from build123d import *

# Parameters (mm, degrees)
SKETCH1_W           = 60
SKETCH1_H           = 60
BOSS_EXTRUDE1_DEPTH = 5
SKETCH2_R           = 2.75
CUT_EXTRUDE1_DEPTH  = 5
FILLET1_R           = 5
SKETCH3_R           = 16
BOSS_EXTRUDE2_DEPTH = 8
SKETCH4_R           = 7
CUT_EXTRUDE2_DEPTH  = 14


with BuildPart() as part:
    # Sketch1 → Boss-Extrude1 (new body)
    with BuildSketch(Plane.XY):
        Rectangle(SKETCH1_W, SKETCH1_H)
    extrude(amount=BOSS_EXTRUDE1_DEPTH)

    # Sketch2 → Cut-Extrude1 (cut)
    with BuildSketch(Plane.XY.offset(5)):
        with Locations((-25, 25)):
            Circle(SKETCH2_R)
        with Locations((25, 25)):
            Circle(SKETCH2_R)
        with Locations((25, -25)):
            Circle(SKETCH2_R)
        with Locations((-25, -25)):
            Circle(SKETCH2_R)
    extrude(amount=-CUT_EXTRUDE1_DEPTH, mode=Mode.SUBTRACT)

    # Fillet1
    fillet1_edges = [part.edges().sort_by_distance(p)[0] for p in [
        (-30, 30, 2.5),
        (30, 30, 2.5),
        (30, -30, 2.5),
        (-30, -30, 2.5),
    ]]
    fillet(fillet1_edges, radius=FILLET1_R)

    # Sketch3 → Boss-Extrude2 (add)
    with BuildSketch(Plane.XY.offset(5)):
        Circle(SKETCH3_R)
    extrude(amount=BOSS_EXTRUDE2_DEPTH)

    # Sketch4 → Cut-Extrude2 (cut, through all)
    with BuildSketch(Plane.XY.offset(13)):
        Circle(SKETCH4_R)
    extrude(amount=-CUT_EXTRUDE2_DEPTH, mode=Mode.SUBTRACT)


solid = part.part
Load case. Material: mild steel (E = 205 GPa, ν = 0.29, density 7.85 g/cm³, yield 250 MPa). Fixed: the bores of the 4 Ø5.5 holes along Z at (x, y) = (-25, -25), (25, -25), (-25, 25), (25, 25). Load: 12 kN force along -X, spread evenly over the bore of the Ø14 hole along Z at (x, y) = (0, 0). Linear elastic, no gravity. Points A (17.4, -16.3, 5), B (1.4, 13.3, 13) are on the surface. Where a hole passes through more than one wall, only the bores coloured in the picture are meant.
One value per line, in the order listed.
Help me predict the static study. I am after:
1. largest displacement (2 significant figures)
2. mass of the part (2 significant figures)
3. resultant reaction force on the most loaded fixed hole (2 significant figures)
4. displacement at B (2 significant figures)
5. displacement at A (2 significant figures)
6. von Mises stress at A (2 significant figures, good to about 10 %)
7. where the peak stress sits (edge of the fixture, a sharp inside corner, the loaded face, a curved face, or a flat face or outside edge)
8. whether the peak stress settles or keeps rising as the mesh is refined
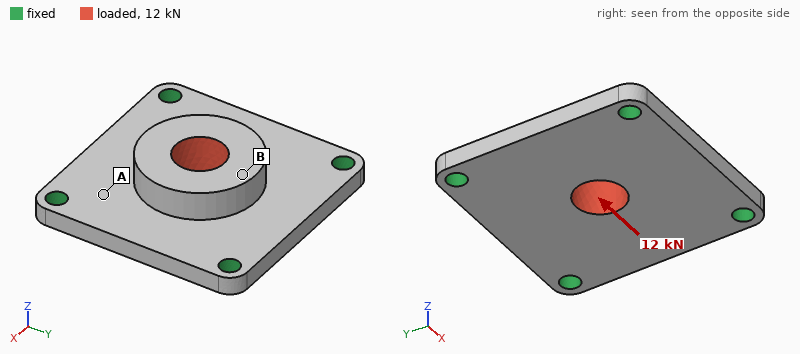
15 µm
170 g
3.4 kN
11 µm
5.0 µm
60 MPa
edge of the fixture
keeps rising
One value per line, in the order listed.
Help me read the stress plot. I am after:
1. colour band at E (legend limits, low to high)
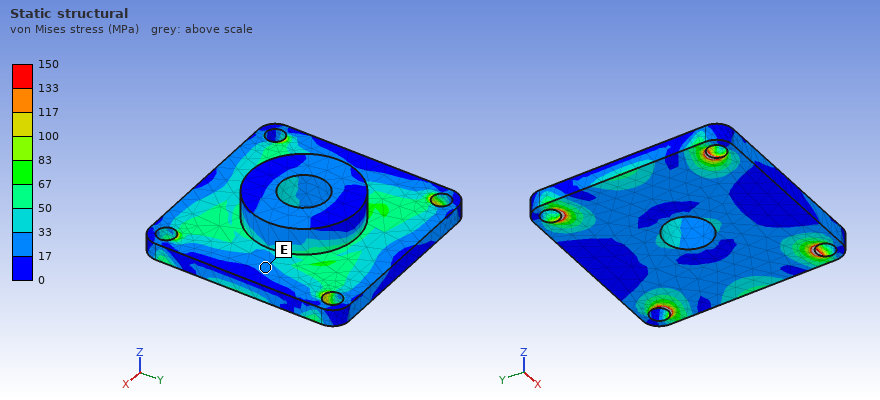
17 to 33 MPa
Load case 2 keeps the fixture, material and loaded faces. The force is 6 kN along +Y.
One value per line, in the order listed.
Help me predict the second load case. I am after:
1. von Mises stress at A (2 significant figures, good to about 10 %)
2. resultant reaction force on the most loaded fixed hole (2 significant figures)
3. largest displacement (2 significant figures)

31 MPa
1.7 kN
7.6 µm
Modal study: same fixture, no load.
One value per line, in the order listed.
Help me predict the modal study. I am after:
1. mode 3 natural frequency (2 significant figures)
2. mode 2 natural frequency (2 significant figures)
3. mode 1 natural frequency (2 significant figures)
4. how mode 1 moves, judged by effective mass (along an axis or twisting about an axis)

11 kHz
11 kHz
7000 Hz
along Z
